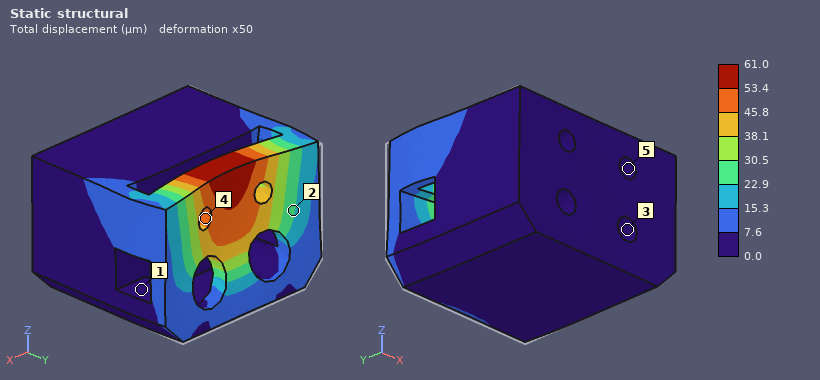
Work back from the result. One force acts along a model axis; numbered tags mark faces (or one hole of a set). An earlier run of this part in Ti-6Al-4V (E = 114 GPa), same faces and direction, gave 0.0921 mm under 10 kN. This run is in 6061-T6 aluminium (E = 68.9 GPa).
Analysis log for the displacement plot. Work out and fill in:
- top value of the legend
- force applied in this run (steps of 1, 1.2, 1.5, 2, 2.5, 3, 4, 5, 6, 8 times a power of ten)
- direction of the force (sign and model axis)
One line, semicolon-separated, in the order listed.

61.0 µm; 4 kN; -Y
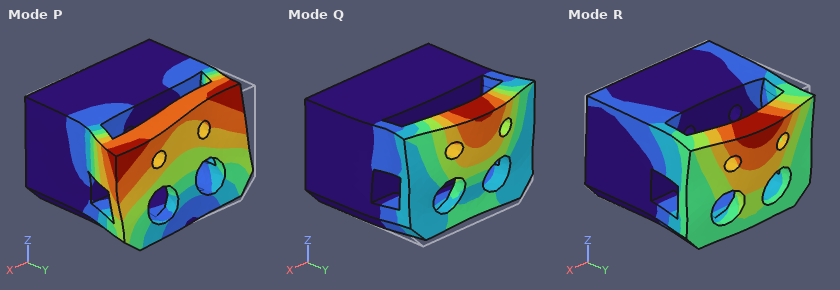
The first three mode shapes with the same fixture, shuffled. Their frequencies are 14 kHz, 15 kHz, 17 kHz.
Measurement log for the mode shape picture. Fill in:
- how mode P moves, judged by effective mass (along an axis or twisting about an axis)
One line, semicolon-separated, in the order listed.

along X
